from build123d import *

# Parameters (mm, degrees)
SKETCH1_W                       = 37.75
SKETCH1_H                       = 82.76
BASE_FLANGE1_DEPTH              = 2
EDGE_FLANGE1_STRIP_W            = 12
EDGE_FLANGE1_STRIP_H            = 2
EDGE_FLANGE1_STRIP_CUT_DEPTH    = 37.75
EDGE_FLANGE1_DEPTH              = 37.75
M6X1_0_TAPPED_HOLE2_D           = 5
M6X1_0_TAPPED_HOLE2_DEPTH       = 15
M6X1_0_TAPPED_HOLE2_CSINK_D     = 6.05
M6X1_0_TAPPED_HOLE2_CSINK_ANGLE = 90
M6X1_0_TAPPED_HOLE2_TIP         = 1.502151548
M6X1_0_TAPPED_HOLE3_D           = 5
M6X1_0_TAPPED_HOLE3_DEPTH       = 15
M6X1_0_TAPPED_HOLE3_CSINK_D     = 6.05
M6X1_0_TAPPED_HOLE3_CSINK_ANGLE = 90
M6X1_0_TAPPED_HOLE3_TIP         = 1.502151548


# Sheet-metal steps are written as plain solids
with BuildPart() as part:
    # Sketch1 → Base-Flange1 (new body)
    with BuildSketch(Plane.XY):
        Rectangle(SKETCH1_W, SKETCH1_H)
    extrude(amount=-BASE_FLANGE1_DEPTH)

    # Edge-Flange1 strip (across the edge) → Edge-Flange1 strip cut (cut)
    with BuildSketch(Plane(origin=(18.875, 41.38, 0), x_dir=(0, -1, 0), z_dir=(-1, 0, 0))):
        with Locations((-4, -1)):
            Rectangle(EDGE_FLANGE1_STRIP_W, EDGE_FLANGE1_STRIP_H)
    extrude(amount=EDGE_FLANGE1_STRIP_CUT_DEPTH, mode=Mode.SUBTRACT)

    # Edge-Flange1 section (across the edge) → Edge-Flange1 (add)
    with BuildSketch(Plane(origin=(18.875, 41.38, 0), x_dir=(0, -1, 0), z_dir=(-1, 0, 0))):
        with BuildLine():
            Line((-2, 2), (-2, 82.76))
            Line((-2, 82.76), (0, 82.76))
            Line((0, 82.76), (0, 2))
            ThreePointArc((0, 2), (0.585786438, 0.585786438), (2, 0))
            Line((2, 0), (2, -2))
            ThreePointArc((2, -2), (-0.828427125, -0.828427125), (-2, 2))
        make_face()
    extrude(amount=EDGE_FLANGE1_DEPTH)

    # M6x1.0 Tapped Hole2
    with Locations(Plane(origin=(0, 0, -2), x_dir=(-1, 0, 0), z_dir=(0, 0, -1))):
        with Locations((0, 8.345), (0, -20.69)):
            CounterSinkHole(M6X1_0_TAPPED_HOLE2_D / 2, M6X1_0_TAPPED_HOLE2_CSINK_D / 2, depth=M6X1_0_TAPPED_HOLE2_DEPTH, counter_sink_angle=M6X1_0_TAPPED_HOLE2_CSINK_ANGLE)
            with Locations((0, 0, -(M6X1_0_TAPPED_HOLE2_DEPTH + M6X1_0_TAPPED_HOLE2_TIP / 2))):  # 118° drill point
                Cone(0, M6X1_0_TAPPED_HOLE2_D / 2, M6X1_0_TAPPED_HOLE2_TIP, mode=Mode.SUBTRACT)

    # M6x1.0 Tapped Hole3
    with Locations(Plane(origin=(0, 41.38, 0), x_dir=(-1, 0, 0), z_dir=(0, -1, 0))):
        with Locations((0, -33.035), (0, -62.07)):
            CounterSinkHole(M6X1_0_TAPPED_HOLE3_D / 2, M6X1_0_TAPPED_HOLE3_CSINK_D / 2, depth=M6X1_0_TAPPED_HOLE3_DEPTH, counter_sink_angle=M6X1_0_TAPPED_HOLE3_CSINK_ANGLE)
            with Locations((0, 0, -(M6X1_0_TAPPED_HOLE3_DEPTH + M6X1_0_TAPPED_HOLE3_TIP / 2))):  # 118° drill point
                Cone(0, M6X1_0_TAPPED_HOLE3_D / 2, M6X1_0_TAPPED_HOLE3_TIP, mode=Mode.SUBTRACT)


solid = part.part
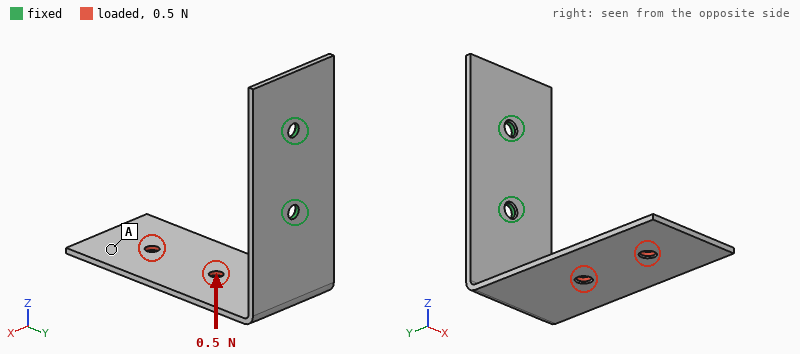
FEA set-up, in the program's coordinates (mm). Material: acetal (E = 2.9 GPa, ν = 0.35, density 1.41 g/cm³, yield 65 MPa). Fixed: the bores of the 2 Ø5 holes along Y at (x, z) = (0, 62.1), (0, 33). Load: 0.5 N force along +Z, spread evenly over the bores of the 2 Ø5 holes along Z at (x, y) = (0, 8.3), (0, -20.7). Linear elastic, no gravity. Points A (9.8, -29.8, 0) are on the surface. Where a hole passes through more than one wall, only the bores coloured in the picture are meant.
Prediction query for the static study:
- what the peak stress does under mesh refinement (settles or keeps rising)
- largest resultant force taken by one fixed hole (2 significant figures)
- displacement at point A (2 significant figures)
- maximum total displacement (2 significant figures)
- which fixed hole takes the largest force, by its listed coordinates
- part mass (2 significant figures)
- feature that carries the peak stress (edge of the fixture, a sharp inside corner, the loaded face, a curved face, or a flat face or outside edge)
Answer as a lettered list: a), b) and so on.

a) keeps rising
b) 0.51 N
c) 1.2 mm
d) 1.4 mm
e) (0, 62.1)
f) 17 g
g) edge of the fixture
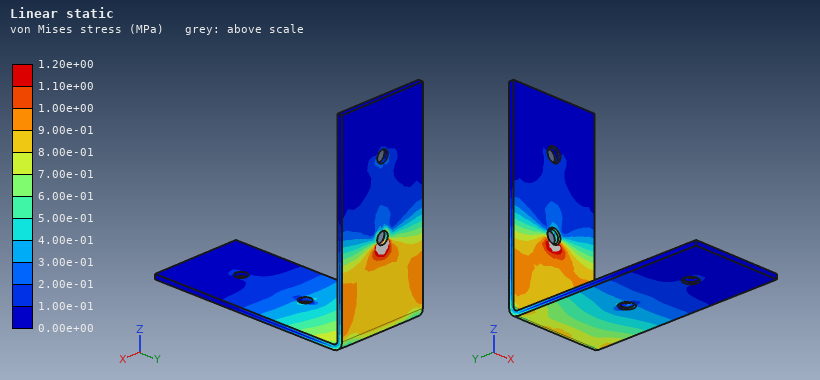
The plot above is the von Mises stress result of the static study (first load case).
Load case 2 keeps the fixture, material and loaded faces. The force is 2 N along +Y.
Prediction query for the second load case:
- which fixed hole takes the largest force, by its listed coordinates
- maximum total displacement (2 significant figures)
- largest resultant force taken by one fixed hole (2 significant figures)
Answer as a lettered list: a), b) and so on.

a) (0, 33)
b) 1.3 mm
c) 2.8 N
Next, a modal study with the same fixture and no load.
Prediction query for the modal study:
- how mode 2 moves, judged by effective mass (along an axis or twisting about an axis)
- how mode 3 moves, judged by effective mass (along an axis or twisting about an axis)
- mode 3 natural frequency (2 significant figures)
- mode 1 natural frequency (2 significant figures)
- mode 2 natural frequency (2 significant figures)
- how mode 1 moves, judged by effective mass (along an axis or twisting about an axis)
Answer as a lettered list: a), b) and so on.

a) along X
b) along Y
c) 160 Hz
d) 41 Hz
e) 64 Hz
f) along Z
